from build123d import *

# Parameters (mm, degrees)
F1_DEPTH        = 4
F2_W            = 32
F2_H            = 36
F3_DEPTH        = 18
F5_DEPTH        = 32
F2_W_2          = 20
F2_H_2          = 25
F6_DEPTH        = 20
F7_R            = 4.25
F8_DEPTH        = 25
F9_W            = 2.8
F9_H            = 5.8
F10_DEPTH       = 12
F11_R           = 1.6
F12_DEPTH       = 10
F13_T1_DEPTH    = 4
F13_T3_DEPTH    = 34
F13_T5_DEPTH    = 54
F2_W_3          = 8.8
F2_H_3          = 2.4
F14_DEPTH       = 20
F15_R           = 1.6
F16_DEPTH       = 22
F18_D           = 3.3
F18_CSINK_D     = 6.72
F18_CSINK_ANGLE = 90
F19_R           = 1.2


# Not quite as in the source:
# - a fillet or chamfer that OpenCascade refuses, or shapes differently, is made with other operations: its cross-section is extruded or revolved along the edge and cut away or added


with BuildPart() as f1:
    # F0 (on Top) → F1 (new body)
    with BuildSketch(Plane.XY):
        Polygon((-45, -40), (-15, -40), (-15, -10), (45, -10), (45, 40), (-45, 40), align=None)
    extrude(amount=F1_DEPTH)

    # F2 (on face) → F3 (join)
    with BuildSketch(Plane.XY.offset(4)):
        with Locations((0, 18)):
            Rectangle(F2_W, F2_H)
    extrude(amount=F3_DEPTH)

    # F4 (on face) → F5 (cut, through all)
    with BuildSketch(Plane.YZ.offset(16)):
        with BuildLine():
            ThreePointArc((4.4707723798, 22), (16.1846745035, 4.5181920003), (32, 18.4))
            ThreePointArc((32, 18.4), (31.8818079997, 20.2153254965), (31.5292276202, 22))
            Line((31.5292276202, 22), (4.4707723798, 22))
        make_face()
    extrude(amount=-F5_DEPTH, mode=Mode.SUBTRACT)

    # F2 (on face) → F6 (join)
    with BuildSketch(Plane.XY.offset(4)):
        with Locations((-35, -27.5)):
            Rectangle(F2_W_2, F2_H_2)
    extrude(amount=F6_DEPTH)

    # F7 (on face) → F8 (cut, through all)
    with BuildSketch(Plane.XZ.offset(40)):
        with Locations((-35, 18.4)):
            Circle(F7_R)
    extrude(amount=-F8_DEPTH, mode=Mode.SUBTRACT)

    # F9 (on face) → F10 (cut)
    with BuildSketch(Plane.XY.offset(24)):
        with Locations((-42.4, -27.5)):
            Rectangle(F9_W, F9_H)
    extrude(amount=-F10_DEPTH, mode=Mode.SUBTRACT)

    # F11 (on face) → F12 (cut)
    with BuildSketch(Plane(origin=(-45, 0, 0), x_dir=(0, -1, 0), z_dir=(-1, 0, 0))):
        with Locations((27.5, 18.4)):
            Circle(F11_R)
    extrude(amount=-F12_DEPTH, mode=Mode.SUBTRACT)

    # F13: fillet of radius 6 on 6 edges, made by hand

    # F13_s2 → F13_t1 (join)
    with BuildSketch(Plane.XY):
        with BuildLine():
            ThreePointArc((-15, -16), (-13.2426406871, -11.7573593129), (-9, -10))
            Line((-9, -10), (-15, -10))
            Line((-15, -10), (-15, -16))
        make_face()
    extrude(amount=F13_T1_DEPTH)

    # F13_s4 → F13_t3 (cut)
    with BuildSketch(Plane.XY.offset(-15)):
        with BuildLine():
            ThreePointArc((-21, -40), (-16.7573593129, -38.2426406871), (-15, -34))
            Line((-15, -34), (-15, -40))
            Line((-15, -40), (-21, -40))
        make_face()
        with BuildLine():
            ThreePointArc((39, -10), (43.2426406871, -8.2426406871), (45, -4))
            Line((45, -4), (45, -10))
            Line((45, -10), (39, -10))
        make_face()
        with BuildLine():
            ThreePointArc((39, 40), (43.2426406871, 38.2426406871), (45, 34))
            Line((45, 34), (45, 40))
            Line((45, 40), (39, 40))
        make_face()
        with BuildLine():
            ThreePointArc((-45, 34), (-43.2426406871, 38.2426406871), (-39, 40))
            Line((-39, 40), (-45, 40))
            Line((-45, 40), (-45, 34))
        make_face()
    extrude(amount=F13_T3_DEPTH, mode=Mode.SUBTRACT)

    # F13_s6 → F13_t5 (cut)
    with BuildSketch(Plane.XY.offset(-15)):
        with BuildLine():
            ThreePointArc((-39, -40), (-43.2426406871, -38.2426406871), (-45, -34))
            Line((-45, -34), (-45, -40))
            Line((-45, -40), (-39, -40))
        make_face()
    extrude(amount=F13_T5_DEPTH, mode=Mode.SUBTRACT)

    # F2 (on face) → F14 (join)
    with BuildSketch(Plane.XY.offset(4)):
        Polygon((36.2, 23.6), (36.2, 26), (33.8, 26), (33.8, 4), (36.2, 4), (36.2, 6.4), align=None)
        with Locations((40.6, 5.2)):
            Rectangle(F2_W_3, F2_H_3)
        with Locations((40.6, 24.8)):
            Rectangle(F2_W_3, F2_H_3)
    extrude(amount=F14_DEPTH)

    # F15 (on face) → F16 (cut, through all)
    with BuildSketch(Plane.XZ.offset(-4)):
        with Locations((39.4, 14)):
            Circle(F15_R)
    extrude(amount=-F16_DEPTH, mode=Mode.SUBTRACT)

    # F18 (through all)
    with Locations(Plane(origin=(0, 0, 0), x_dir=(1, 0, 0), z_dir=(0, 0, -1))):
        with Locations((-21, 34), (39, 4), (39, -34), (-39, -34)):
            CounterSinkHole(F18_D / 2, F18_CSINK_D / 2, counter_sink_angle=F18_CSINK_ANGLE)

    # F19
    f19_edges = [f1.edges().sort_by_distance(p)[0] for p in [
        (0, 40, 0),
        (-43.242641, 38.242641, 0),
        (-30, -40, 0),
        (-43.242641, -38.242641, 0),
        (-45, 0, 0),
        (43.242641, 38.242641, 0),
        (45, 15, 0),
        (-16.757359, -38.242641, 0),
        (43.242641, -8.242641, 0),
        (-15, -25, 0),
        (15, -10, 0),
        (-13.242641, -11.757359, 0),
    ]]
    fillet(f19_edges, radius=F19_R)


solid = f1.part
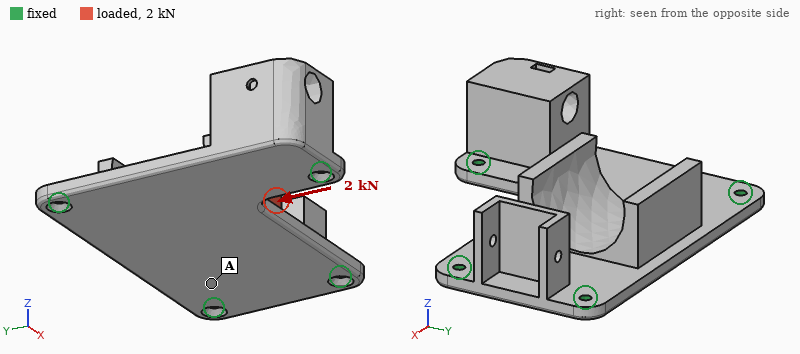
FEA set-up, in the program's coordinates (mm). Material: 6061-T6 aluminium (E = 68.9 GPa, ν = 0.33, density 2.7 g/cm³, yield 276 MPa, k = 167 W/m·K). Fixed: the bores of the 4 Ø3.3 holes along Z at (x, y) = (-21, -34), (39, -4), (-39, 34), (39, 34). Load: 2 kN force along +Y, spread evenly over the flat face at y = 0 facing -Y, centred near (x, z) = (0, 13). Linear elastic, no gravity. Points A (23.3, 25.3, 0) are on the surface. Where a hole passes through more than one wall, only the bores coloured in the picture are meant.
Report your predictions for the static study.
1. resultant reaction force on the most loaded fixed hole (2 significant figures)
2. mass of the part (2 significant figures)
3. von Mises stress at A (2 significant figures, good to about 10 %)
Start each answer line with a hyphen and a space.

- 700 N
- 110 g
- 13 MPa
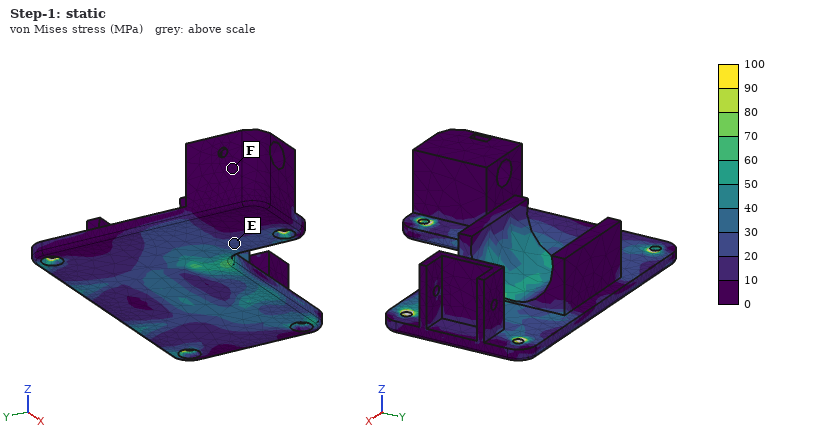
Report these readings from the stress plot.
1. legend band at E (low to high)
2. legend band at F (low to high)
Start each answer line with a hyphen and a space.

- 20 to 30 MPa
- 0 to 10 MPa
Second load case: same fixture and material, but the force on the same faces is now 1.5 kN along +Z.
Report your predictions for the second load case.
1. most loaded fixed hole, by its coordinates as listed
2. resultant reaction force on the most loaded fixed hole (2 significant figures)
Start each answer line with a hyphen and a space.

- (39, -4)
- 630 N
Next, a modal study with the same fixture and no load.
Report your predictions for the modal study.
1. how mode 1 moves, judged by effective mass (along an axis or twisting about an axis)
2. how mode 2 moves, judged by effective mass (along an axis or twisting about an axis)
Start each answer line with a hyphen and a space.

- along Z
- along Z
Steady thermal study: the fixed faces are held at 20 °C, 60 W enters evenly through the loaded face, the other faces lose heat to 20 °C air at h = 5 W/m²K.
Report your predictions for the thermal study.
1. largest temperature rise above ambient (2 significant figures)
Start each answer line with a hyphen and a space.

- 56 K
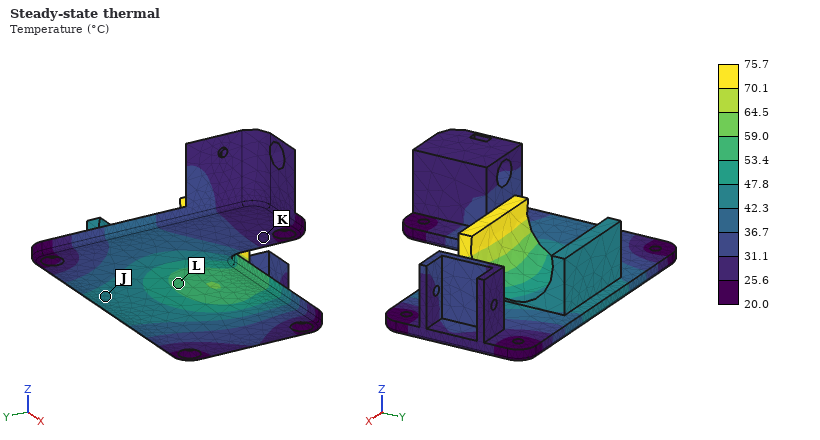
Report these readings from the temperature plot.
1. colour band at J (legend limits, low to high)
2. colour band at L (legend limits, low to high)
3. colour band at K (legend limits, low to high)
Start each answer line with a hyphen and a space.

- 42.3 to 47.8 °C
- 53.4 to 59.0 °C
- 25.6 to 31.1 °C
